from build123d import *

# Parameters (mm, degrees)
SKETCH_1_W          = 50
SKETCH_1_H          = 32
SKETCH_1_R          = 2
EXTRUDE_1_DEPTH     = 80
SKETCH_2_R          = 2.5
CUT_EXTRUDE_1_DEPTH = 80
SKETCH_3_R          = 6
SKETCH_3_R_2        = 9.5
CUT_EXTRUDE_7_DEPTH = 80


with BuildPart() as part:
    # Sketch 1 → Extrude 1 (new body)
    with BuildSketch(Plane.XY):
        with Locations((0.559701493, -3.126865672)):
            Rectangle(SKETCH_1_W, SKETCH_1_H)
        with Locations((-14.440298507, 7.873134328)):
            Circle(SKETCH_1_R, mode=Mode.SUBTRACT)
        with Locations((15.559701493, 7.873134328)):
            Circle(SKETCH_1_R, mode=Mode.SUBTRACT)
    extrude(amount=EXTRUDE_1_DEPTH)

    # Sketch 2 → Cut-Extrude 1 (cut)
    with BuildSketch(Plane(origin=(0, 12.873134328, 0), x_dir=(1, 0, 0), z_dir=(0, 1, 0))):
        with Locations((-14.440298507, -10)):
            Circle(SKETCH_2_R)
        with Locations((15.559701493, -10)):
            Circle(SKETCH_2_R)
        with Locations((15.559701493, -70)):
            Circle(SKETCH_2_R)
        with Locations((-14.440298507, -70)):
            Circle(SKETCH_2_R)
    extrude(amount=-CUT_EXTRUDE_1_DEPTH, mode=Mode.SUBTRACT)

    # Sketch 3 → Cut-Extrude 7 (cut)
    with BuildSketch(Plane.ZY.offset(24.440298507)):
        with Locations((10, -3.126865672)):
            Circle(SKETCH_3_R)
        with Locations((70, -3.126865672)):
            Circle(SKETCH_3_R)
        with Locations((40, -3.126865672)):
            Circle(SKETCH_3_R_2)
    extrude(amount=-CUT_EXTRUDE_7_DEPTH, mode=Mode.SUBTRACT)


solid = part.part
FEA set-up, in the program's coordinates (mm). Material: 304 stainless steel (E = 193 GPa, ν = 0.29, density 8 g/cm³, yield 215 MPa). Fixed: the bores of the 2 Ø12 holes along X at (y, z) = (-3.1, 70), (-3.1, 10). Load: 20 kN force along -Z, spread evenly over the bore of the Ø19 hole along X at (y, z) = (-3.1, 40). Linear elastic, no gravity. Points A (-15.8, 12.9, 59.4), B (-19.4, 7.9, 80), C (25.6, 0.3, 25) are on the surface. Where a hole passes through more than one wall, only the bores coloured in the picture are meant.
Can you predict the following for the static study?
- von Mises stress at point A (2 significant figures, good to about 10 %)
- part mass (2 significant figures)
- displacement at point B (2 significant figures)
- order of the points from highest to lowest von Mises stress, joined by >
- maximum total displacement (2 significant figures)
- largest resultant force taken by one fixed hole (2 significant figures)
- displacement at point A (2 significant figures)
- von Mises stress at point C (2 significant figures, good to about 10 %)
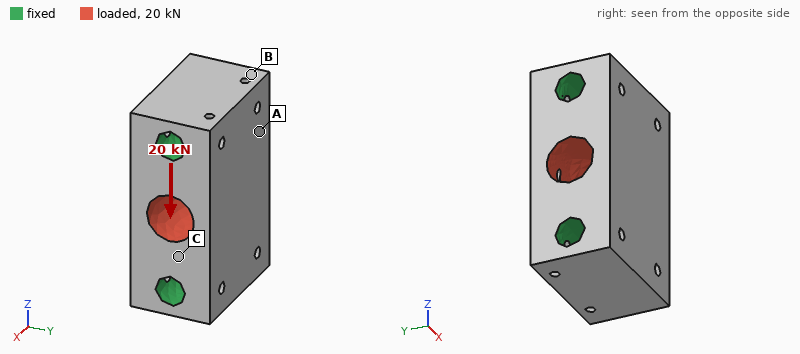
2.8 MPa
790 g
0.25 µm
C > A > B
1.2 µm
10 kN
0.55 µm
8.9 MPa
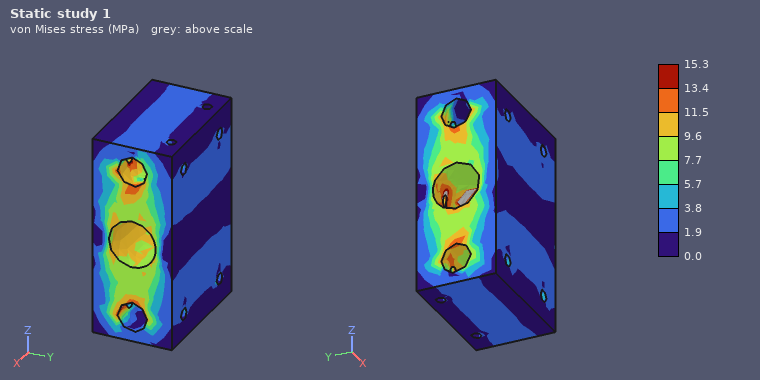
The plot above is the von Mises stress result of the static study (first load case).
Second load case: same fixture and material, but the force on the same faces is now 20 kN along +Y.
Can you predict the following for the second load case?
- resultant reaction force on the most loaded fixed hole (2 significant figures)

10 kN
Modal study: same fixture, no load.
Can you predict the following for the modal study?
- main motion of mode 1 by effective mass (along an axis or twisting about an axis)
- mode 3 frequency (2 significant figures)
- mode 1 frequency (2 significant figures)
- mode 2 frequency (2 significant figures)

along Y
28 kHz
24 kHz
27 kHz
